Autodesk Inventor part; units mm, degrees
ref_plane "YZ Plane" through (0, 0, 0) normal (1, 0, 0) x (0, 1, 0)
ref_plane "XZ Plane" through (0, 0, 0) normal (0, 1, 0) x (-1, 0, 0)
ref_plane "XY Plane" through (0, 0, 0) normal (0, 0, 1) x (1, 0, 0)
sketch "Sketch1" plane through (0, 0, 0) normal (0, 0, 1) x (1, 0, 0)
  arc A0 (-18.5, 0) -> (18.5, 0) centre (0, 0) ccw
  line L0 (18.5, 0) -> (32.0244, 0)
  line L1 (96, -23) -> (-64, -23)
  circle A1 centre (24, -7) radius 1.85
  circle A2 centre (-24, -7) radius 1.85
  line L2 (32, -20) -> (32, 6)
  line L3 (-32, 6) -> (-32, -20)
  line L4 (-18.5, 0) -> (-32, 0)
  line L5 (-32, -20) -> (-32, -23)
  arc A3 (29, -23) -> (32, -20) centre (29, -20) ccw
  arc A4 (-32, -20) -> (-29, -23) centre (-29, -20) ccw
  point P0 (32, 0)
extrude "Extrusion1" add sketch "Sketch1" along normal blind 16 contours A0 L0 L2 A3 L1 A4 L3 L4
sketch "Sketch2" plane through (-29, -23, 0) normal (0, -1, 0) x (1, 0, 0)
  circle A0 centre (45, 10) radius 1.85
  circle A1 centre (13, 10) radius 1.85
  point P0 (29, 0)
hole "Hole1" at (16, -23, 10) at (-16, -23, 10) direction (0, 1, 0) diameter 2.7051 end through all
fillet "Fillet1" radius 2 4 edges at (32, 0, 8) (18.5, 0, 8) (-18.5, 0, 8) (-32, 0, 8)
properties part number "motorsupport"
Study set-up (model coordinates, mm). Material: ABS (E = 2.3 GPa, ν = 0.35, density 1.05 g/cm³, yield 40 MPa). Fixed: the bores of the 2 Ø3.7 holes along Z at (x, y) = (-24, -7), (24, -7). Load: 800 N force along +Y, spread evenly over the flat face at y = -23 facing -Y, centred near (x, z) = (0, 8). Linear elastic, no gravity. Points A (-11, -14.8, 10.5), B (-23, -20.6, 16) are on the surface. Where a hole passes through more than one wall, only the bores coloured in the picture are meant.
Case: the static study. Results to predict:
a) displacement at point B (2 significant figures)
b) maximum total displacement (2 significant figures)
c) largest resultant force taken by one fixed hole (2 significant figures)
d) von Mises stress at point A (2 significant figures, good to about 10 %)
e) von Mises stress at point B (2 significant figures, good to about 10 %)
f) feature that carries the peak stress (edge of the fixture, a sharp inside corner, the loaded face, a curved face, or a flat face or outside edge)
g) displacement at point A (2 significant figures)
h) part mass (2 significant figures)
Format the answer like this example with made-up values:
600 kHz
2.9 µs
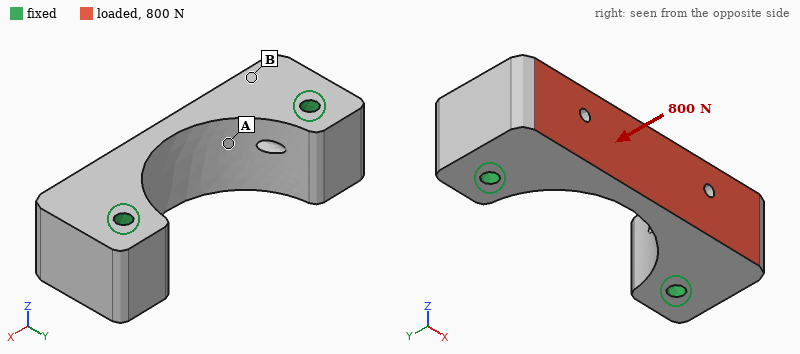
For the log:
13 µm
78 µm
460 N
4.4 MPa
1.1 MPa
a curved face
39 µm
15 g
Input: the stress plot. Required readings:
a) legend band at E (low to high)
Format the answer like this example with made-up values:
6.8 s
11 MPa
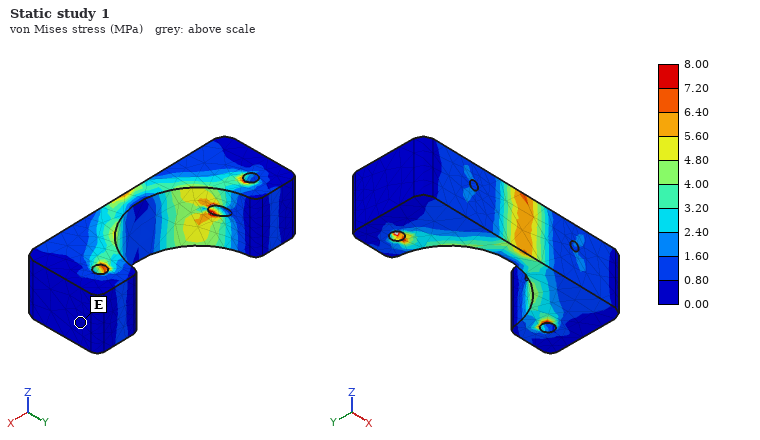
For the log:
0.00 to 0.80 MPa
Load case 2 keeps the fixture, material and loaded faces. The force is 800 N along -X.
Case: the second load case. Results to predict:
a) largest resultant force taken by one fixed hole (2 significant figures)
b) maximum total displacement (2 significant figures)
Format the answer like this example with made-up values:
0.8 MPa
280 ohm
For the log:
430 N
0.10 mm
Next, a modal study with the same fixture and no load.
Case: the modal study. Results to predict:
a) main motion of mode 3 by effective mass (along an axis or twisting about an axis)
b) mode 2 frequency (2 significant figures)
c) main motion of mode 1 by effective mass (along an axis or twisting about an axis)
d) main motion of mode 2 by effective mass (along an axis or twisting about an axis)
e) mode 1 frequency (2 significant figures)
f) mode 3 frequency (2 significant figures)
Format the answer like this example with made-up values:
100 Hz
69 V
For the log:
along Y
5400 Hz
along X
along Z
5100 Hz
7600 Hz
